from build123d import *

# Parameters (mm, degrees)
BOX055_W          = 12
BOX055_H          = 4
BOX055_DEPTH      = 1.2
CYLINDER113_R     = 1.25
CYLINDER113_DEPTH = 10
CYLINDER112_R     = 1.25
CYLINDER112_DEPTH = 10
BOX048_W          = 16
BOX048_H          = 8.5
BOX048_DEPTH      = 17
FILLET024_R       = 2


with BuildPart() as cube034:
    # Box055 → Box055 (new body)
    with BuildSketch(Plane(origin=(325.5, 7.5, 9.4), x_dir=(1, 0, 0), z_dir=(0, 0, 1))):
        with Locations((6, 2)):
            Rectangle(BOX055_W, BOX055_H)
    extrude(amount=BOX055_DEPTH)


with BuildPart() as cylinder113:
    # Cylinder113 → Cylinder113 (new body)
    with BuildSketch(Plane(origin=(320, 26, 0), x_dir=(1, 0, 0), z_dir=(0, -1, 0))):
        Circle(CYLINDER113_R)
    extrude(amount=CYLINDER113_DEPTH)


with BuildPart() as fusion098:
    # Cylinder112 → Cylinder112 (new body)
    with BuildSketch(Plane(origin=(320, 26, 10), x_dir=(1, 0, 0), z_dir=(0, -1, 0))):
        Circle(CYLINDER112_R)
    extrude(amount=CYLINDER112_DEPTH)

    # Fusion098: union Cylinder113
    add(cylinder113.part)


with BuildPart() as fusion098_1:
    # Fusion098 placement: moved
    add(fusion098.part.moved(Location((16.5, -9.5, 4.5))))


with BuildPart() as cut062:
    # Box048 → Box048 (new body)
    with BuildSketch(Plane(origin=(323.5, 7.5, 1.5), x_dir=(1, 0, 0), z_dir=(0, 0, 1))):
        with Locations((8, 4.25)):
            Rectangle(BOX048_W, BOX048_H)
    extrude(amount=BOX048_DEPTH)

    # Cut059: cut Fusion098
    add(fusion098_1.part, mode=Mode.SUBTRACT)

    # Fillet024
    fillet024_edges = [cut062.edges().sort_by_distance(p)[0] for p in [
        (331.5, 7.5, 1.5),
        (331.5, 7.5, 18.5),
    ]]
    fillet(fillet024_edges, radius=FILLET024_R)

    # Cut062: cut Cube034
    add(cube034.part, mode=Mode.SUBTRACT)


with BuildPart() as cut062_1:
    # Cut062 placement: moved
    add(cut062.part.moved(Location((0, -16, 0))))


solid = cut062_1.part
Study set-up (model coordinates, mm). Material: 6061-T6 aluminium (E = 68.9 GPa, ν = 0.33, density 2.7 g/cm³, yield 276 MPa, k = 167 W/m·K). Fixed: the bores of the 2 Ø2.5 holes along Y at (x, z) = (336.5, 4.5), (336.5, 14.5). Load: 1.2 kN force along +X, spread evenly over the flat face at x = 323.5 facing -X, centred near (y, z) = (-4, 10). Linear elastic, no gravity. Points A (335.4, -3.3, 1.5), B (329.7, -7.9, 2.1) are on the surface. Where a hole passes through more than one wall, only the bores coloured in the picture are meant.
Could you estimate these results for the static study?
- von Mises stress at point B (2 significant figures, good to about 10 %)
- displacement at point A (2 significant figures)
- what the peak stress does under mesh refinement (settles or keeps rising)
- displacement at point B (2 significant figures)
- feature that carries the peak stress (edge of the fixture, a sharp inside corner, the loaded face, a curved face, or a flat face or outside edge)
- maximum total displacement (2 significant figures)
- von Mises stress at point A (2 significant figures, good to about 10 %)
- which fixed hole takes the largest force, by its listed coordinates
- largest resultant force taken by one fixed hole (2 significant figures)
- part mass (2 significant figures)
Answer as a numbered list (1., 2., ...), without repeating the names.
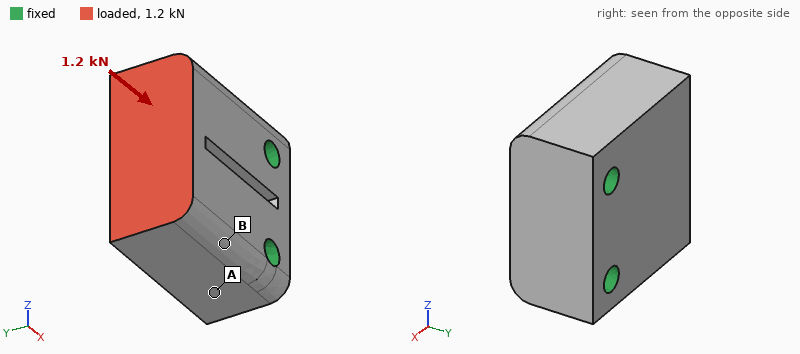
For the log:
1. 8.9 MPa
2. 0.30 µm
3. keeps rising
4. 0.94 µm
5. edge of the fixture
6. 1.9 µm
7. 4.6 MPa
8. (336.5, 14.5)
9. 650 N
10. 5.8 g
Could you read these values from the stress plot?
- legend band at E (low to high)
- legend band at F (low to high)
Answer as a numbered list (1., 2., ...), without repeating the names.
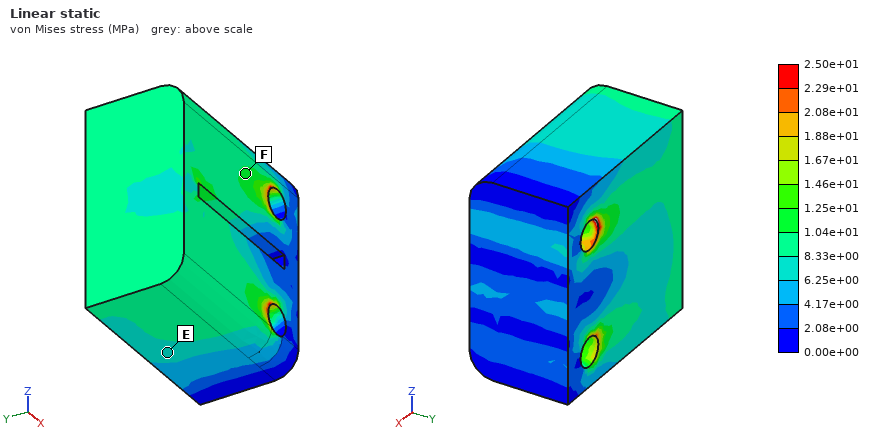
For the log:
1. 6.25e+00 to 8.33e+00 MPa
2. 1.04e+01 to 1.25e+01 MPa
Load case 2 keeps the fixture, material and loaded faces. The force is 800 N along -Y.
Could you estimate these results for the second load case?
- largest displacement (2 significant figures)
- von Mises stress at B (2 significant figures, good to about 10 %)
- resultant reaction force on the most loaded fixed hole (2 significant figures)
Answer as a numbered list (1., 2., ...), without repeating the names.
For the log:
1. 16 µm
2. 25 MPa
3. 420 N
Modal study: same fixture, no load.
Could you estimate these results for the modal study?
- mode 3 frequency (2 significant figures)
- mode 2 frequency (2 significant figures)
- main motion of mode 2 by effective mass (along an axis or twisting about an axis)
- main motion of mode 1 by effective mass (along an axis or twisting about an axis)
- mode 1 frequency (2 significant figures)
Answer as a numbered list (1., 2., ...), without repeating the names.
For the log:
1. 48 kHz
2. 39 kHz
3. along Z
4. along Y
5. 31 kHz
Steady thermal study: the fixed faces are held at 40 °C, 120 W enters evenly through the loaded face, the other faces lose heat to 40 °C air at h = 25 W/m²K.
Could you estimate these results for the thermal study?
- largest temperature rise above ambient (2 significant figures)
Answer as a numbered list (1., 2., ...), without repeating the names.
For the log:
1. 68 K
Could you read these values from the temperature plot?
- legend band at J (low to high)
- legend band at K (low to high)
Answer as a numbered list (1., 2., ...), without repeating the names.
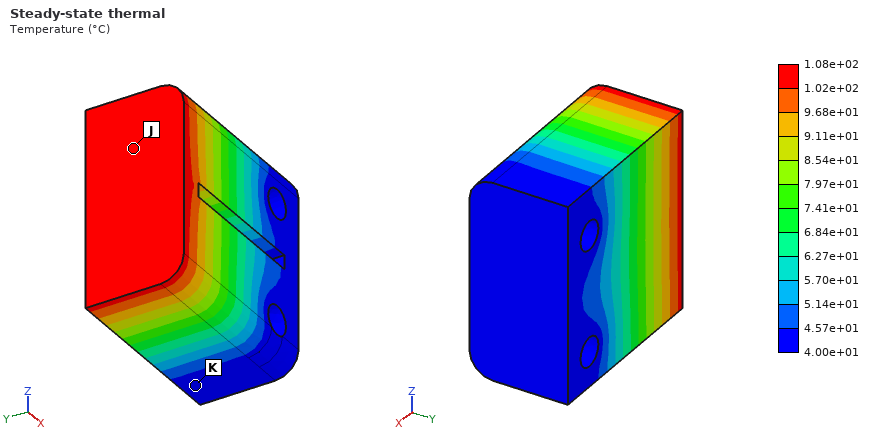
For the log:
1. 1.02e+02 to 1.08e+02 °C
2. 4.00e+01 to 4.57e+01 °C
